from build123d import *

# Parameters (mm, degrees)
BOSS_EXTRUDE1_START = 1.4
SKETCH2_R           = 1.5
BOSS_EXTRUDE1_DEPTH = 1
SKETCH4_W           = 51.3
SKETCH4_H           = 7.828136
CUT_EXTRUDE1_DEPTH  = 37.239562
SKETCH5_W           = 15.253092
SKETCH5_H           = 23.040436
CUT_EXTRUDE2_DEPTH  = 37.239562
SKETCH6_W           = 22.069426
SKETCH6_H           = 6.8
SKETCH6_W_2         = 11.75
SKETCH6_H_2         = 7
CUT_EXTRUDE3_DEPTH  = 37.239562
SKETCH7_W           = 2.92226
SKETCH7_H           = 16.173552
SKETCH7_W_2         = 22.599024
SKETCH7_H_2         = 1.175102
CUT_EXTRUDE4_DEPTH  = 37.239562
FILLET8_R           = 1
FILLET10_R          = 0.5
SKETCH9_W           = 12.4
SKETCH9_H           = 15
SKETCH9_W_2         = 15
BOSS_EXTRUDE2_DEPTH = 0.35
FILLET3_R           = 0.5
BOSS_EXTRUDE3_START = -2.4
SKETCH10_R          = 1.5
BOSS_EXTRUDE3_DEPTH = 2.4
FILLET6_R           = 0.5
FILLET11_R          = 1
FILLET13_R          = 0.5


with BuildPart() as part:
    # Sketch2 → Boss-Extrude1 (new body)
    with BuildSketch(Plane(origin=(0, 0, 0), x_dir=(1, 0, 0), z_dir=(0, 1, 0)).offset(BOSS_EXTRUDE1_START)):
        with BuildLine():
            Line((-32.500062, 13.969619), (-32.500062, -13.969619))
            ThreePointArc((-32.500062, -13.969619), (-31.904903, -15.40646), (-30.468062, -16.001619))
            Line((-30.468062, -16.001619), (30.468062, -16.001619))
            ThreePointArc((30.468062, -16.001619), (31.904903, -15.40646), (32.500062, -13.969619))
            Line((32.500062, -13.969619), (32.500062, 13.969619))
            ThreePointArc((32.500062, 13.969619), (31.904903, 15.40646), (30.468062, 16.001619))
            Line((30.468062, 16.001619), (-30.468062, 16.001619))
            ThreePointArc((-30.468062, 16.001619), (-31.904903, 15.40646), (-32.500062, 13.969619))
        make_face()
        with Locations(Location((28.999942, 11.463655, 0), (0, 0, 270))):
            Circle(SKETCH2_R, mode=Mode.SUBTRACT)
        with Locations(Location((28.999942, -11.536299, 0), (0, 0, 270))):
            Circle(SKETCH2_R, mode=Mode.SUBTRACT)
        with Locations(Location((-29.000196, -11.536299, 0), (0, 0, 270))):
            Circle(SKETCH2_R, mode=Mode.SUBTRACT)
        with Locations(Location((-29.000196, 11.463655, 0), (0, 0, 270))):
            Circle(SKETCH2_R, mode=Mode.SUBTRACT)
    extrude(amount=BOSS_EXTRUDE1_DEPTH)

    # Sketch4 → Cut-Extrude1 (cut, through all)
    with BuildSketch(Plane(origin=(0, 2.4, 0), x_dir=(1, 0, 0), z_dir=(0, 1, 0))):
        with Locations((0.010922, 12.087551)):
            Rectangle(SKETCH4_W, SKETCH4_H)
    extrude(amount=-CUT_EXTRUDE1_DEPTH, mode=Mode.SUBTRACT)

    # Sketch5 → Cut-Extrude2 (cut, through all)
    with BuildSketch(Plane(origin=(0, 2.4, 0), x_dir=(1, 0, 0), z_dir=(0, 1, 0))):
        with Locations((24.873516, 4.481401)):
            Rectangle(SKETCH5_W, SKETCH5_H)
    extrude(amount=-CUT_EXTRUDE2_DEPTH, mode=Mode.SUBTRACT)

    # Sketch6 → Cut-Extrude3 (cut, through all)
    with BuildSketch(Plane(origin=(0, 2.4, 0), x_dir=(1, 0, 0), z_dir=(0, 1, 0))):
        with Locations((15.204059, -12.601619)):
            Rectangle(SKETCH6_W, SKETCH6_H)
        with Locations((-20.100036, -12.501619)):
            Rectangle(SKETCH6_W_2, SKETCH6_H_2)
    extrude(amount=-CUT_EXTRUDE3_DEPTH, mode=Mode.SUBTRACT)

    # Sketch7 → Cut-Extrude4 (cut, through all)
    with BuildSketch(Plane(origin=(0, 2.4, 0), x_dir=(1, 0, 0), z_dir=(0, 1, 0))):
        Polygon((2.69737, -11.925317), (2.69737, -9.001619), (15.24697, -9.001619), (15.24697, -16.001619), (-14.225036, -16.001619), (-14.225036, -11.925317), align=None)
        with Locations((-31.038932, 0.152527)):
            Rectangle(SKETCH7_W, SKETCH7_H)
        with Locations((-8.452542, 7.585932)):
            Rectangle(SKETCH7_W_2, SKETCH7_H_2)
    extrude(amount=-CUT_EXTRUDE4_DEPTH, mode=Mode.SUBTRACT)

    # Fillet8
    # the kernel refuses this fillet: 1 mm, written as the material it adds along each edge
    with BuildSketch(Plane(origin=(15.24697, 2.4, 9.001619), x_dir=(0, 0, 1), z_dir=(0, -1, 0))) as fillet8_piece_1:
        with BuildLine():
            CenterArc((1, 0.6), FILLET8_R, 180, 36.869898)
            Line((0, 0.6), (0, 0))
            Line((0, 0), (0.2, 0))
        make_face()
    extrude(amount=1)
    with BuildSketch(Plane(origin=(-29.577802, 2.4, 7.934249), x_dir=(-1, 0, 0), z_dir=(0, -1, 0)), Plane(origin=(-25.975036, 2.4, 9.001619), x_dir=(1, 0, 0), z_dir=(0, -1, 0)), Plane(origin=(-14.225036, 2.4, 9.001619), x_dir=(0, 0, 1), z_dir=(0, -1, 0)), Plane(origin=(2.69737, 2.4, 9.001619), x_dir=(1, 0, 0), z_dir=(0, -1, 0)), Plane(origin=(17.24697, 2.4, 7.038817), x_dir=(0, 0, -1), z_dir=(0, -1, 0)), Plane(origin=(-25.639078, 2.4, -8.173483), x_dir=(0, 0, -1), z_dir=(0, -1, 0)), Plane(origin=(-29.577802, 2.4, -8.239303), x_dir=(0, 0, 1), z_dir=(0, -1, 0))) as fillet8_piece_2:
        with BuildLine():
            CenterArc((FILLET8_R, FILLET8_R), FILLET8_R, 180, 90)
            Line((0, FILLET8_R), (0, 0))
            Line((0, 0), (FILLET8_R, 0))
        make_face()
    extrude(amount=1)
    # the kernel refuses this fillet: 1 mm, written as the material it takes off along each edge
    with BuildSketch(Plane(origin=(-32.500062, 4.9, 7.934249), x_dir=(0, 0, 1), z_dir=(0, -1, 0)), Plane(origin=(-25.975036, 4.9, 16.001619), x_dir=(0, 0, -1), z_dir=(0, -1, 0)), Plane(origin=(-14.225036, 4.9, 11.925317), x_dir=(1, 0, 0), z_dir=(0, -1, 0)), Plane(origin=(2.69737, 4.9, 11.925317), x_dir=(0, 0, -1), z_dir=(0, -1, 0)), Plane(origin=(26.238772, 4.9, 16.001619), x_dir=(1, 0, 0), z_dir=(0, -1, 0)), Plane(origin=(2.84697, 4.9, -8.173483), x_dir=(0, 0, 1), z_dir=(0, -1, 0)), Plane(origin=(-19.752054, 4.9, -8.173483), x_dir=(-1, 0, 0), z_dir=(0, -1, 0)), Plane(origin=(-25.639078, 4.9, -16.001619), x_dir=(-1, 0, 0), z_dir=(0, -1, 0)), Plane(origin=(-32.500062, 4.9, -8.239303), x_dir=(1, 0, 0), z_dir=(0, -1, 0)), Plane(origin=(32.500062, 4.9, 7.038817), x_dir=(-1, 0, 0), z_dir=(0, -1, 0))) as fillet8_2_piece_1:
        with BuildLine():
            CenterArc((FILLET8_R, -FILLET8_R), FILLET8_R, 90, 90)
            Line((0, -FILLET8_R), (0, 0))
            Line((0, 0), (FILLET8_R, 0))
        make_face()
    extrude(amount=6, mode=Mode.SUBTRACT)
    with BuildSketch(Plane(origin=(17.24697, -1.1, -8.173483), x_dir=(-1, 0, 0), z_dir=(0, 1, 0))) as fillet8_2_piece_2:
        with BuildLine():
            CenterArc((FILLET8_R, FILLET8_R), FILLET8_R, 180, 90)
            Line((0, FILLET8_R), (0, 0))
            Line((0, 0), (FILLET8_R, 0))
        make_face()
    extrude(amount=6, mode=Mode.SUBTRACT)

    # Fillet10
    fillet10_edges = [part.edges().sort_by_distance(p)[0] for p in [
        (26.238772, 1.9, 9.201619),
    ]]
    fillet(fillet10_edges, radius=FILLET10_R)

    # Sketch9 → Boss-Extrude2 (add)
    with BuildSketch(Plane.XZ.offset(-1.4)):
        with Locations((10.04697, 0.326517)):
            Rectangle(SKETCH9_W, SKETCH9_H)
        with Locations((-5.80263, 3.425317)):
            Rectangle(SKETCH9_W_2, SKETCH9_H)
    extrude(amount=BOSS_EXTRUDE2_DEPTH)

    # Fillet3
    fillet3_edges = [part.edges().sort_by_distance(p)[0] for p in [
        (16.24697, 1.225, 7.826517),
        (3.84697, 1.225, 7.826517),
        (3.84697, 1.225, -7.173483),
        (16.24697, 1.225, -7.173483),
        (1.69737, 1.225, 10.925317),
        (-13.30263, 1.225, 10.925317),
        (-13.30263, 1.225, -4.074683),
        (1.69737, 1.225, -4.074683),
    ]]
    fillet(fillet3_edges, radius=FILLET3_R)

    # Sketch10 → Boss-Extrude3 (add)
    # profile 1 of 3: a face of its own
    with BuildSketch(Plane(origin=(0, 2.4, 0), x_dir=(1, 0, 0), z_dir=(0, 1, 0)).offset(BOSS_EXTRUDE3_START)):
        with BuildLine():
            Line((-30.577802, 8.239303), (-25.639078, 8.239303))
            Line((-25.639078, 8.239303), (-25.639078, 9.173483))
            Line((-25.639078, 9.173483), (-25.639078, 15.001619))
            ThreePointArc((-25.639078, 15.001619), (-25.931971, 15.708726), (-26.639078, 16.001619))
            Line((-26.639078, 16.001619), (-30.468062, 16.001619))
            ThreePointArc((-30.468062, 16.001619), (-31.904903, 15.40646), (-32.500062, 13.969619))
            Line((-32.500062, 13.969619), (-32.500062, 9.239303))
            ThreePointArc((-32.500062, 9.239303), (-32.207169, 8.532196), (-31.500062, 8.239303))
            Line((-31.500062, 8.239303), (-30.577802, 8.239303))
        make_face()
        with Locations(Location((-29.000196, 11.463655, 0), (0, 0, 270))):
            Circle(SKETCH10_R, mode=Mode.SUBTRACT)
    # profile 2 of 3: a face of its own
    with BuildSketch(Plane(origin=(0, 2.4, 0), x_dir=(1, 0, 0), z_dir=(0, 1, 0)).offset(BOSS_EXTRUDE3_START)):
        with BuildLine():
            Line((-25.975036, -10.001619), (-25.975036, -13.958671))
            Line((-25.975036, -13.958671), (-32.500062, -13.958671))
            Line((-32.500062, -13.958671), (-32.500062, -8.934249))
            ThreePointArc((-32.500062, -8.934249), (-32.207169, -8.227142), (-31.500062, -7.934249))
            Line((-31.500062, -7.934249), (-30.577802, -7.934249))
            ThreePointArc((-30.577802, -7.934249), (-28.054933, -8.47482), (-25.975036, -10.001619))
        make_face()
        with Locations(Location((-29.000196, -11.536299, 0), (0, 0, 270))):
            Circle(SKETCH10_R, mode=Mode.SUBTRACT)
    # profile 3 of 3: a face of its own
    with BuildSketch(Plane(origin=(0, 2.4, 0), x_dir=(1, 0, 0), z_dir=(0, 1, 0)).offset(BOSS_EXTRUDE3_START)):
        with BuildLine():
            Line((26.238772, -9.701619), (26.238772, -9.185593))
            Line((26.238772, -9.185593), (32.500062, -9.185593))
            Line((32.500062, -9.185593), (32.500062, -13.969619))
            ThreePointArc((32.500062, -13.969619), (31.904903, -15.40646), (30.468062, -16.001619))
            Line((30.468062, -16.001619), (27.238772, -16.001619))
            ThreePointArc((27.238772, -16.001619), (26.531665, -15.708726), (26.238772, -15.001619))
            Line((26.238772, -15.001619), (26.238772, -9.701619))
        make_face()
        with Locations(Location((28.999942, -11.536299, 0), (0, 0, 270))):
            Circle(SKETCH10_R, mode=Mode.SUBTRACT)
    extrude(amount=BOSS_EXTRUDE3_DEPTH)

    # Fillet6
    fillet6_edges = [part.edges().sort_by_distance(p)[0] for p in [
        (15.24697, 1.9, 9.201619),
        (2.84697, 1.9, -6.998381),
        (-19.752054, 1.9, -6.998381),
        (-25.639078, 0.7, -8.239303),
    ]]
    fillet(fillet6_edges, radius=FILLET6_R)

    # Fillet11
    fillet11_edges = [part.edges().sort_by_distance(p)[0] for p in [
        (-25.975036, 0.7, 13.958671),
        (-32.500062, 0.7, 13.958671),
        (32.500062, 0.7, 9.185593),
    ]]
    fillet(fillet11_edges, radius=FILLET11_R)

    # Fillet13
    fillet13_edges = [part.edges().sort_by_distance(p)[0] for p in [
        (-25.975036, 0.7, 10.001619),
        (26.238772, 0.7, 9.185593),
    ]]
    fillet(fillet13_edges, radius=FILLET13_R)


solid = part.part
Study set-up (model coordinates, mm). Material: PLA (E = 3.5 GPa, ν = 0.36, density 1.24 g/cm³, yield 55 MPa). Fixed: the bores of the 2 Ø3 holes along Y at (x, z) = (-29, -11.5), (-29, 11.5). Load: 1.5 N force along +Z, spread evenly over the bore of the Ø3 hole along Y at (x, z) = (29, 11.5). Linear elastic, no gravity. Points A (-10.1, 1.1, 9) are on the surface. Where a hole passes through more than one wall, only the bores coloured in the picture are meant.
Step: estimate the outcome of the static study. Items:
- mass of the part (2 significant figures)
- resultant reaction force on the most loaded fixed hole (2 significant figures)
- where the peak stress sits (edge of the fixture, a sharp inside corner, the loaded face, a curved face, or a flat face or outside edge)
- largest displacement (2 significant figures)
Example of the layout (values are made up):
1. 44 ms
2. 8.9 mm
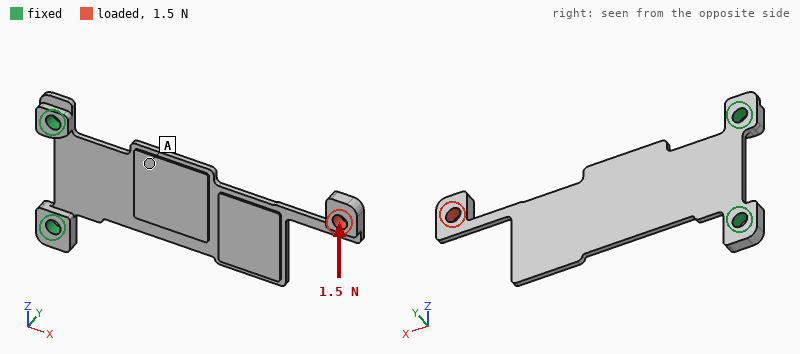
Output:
1. 1.6 g
2. 4.9 N
3. a curved face
4. 0.69 mm
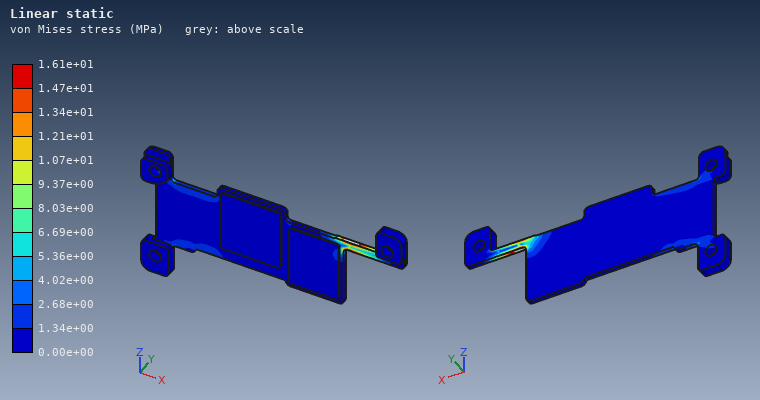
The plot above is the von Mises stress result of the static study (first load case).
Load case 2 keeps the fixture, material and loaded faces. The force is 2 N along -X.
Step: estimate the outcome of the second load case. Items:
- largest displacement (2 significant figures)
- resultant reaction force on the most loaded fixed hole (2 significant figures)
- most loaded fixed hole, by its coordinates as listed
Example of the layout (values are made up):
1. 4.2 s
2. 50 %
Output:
1. 0.75 mm
2. 2.4 N
3. (-29, 11.5)
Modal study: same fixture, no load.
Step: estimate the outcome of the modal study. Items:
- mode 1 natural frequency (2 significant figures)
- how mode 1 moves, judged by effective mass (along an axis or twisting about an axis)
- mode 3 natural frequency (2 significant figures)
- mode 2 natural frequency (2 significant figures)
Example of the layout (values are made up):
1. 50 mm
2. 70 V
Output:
1. 84 Hz
2. along Y
3. 690 Hz
4. 340 Hz
